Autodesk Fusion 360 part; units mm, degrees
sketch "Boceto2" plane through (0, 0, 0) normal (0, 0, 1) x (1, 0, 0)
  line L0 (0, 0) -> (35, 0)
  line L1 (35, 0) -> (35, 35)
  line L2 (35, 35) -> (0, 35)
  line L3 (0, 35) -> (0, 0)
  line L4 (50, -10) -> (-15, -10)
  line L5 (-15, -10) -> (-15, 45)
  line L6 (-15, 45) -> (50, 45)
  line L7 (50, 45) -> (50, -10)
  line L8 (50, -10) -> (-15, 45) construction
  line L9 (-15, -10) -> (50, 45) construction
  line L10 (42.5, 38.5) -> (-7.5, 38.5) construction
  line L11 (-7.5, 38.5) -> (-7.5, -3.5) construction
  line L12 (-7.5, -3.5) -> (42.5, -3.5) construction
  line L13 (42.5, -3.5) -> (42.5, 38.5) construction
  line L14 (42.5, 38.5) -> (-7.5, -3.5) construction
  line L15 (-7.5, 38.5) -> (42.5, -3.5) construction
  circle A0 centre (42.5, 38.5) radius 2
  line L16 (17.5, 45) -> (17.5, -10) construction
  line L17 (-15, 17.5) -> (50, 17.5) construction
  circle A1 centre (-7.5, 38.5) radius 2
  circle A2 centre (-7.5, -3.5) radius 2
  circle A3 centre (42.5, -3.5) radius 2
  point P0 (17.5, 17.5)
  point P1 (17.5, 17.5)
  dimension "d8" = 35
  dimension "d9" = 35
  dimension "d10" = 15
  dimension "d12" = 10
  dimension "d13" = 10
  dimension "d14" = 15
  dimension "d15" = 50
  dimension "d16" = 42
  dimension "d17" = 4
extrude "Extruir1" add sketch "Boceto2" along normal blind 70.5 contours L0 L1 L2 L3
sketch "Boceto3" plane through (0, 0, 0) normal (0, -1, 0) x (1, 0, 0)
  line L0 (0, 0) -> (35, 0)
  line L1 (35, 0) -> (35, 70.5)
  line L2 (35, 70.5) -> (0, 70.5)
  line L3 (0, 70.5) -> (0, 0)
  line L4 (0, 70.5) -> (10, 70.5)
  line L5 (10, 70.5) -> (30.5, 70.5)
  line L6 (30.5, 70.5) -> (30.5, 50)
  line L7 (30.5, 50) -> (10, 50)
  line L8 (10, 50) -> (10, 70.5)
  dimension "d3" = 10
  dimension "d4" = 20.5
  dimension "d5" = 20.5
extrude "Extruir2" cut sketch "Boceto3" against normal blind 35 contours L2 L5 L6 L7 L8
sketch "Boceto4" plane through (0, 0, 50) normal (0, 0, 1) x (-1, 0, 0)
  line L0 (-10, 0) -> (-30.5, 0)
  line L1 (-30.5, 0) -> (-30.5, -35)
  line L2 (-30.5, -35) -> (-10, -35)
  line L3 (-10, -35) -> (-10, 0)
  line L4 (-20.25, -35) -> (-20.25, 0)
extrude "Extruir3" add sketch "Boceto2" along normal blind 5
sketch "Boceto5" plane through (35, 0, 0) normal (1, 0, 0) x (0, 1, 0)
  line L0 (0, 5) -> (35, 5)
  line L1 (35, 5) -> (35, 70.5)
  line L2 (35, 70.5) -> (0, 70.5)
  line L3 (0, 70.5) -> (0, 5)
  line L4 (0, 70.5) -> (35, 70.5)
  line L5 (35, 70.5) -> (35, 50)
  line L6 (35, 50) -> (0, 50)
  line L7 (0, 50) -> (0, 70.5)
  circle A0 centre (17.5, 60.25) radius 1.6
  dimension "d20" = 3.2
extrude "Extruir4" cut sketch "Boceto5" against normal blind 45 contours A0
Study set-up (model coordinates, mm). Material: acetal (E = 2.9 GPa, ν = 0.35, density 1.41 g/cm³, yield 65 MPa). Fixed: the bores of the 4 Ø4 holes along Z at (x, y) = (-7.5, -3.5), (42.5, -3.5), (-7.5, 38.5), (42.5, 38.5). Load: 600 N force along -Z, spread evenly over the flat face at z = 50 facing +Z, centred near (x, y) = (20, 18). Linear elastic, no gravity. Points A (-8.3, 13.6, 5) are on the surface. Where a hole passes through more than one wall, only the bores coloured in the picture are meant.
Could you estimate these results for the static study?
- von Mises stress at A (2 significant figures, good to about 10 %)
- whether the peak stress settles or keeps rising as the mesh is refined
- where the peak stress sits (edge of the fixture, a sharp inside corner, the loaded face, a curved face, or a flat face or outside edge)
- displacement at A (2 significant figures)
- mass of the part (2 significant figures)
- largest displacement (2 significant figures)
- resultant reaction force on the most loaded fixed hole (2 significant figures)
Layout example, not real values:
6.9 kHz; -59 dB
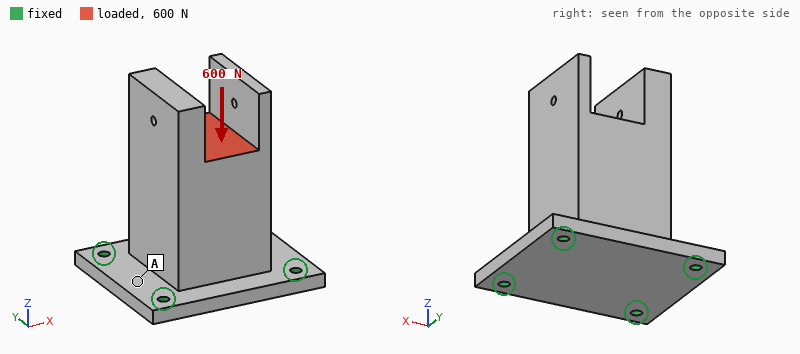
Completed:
1.6 MPa; keeps rising; edge of the fixture; 39 µm; 120 g; 92 µm; 180 N
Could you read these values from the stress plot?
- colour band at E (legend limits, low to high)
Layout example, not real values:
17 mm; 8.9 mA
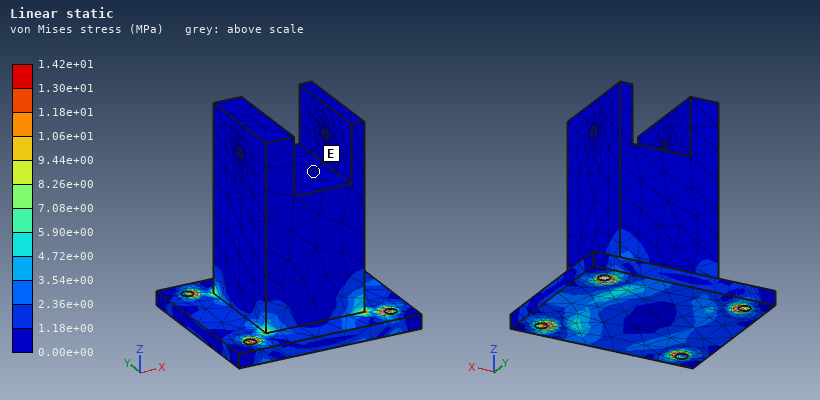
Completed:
0.00e+00 to 1.18e+00 MPa
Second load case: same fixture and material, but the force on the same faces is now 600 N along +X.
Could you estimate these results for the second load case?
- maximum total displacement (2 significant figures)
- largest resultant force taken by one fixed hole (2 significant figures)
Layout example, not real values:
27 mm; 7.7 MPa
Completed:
0.63 mm; 370 N
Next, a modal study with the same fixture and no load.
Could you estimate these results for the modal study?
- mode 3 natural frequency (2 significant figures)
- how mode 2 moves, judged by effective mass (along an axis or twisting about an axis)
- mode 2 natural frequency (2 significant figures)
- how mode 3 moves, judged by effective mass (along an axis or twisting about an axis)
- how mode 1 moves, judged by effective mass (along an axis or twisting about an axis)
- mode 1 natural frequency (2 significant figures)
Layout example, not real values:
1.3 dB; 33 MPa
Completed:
1400 Hz; along X; 810 Hz; along Z; along Y; 720 Hz
